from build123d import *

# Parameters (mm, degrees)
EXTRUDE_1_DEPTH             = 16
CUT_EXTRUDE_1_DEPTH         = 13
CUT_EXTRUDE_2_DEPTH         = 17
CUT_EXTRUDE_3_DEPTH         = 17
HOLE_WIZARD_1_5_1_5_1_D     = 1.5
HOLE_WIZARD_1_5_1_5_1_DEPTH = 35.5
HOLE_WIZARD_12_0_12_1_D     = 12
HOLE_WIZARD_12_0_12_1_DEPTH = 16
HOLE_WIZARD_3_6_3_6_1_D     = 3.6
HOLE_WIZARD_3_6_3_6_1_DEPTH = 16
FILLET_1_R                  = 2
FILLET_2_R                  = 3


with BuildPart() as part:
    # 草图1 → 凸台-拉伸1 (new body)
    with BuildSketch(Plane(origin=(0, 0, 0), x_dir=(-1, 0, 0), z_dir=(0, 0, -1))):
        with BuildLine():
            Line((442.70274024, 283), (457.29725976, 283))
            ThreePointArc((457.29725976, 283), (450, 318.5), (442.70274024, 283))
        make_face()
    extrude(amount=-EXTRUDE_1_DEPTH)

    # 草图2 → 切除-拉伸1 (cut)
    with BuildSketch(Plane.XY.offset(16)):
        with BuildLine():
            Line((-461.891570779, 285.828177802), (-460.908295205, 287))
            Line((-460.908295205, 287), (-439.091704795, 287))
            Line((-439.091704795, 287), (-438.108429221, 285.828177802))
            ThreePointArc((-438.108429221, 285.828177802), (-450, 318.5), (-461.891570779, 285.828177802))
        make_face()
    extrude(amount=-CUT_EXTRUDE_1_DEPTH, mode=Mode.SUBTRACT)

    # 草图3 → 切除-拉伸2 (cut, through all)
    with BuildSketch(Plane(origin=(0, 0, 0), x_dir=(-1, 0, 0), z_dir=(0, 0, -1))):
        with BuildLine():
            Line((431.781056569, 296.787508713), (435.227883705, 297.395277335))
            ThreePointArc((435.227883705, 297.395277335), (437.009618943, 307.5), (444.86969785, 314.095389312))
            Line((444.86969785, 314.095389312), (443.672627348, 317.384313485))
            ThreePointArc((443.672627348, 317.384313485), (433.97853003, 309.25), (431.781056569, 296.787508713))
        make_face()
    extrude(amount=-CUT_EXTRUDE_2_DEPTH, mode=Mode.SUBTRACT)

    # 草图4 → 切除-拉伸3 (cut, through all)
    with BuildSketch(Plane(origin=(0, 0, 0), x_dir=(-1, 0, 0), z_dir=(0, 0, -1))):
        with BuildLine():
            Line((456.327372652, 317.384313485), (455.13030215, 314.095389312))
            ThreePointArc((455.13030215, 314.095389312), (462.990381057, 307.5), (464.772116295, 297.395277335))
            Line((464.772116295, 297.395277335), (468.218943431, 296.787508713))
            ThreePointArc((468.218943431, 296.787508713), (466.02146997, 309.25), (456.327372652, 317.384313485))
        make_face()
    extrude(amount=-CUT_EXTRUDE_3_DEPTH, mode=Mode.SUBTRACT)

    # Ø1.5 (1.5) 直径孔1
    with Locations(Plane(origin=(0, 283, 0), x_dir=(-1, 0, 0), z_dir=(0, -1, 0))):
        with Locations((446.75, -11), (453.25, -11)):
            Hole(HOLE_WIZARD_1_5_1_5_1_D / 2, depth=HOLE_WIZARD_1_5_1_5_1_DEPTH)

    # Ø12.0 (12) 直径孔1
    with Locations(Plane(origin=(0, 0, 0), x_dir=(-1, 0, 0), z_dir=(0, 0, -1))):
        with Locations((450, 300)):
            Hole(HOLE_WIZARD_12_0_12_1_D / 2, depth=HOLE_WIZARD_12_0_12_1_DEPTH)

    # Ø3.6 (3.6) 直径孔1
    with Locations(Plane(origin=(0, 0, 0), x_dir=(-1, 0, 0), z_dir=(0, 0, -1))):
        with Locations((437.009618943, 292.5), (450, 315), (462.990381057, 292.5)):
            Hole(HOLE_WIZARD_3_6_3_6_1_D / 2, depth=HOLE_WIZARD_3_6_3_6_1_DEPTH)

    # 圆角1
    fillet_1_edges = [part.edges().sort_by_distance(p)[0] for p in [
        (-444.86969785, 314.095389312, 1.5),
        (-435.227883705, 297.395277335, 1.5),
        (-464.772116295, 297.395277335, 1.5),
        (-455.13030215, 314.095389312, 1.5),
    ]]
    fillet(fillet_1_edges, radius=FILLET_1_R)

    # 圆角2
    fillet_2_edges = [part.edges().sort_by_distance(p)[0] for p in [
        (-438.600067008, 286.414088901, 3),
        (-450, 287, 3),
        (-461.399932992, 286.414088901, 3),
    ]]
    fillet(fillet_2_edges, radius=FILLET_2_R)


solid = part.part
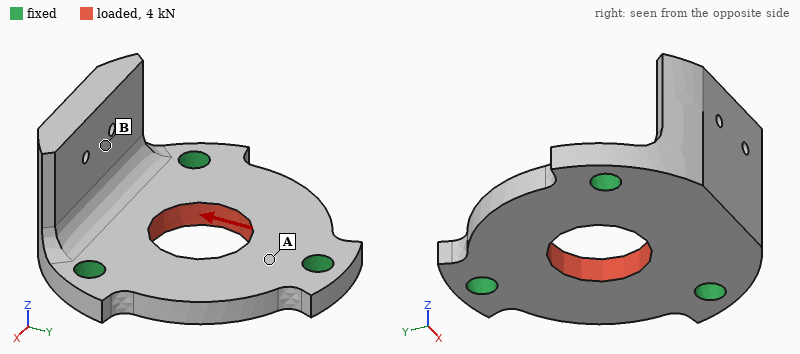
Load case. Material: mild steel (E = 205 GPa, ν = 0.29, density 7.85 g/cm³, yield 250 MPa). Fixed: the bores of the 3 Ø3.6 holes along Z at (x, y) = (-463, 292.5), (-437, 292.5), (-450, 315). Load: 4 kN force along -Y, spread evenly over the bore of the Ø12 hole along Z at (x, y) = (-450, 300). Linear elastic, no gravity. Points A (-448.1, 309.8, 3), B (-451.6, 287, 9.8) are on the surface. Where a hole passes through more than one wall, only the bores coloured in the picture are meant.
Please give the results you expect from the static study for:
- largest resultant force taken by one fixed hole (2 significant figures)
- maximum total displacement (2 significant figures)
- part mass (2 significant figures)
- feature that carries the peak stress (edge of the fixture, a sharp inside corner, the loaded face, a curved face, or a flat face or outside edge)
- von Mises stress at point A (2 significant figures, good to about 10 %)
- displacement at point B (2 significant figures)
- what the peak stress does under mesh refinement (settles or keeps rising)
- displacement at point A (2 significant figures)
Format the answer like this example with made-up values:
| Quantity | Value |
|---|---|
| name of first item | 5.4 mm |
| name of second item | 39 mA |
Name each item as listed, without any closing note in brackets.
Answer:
| Quantity | Value |
|---|---|
| largest resultant force taken by one fixed hole | 1.4 kN |
| maximum total displacement | 4.4 µm |
| part mass | 26 g |
| feature that carries the peak stress | edge of the fixture |
| von Mises stress at point A | 54 MPa |
| displacement at point B | 3.3 µm |
| what the peak stress does under mesh refinement | keeps rising |
| displacement at point A | 1.1 µm |
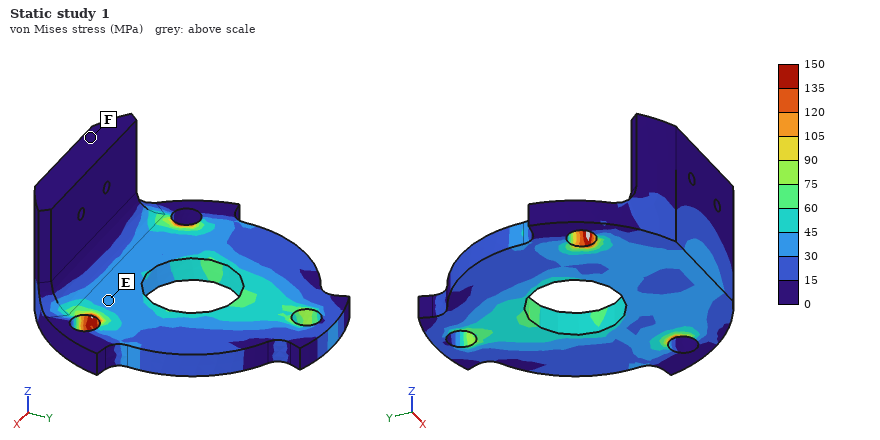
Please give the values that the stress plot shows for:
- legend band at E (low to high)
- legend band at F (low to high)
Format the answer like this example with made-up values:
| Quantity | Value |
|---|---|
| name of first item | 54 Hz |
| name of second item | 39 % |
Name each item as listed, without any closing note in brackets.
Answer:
| Quantity | Value |
|---|---|
| legend band at E | 30 to 45 MPa |
| legend band at F | 0 to 15 MPa |
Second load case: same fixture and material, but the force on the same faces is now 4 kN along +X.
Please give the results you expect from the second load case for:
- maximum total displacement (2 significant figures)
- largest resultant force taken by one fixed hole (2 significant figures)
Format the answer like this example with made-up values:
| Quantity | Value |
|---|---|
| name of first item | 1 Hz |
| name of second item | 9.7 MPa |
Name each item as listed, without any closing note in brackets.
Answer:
| Quantity | Value |
|---|---|
| maximum total displacement | 5.1 µm |
| largest resultant force taken by one fixed hole | 1.3 kN |
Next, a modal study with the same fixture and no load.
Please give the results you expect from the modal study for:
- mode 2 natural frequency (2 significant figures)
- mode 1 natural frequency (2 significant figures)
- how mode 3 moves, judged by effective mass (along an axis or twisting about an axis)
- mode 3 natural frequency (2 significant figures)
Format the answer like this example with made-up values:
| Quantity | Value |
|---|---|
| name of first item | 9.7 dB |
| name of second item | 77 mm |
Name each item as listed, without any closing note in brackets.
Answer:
| Quantity | Value |
|---|---|
| mode 2 natural frequency | 19 kHz |
| mode 1 natural frequency | 7100 Hz |
| how mode 3 moves, judged by effective mass | along Z |
| mode 3 natural frequency | 21 kHz |
